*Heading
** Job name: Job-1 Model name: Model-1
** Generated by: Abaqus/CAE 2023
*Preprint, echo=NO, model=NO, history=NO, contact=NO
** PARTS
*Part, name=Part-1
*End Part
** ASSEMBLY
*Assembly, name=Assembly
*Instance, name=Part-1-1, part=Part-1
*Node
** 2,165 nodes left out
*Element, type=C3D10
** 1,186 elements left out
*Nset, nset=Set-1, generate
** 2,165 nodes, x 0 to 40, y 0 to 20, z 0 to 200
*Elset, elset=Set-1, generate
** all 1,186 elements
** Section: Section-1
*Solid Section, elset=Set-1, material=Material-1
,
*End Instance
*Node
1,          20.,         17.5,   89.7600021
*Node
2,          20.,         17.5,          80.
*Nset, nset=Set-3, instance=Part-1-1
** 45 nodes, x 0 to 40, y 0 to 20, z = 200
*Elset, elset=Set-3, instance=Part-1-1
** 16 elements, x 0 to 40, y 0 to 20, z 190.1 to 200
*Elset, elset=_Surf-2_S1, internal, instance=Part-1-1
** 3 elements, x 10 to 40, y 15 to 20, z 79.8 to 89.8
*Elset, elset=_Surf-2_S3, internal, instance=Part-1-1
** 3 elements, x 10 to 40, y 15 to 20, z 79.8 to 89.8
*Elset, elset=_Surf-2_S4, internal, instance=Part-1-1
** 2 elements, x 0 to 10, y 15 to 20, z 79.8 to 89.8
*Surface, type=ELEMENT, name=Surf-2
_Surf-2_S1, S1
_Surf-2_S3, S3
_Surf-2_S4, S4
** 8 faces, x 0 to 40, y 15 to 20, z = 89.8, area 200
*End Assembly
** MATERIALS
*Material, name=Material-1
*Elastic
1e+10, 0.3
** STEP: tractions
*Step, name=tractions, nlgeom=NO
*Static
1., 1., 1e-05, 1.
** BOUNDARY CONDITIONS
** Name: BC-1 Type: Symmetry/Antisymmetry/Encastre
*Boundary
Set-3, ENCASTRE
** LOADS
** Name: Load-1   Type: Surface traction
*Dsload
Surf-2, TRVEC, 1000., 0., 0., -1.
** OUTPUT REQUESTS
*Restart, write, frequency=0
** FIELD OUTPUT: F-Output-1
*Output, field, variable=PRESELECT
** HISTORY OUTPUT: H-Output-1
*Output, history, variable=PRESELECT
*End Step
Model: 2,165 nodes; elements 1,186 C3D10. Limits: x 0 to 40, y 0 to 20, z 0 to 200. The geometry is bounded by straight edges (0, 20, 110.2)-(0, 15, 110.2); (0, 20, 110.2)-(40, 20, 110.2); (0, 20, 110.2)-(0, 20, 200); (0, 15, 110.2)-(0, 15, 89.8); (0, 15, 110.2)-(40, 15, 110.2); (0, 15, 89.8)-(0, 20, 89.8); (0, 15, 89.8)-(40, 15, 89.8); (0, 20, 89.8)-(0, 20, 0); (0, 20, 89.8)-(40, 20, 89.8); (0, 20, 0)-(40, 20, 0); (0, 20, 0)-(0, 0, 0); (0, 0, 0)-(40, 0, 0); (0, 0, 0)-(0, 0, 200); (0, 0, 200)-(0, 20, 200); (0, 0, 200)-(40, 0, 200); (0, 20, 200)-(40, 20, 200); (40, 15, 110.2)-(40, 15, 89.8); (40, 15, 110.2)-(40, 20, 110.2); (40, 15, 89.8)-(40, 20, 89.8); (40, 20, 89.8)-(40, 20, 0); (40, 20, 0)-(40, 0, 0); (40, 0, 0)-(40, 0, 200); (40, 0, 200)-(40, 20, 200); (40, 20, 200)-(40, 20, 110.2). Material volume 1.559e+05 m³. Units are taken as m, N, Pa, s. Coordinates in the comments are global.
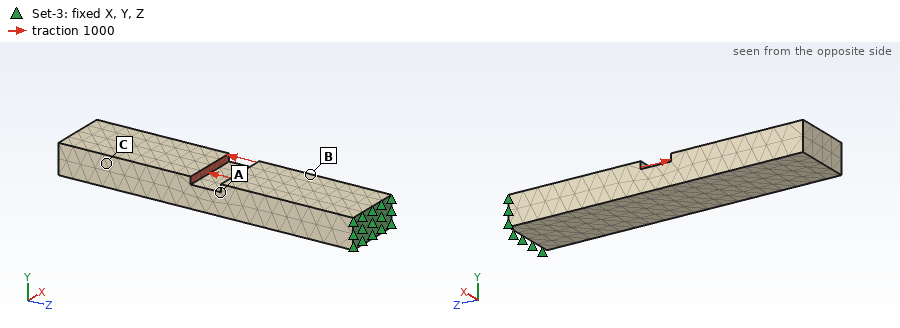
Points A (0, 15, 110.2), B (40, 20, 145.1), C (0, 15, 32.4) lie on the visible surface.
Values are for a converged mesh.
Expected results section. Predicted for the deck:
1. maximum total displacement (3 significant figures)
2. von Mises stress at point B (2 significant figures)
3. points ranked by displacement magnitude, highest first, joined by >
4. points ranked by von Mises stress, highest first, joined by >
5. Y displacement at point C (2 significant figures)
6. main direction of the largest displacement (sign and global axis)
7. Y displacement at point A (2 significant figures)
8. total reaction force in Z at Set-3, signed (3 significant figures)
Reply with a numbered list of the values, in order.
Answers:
1. 1.25e-04 m
2. 810 Pa
3. C > A > B
4. A > B > C
5. -9.3e-05 m
6. -Y
7. -2.2e-05 m
8. 2.00e+05 N
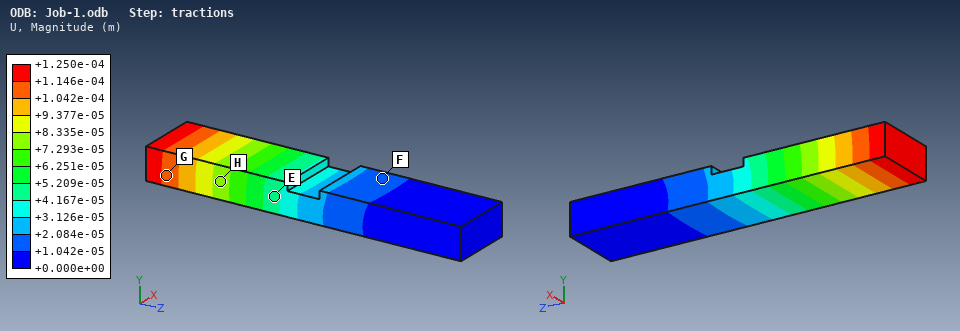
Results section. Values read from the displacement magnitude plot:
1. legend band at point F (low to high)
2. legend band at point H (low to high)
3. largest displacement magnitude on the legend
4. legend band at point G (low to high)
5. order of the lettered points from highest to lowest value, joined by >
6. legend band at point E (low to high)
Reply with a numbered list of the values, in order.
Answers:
1. +1.042e-05 to +2.084e-05 m
2. +7.293e-05 to +8.335e-05 m
3. +1.250e-04 m
4. +1.042e-04 to +1.146e-04 m
5. G > H > E > F
6. +4.167e-05 to +5.209e-05 m
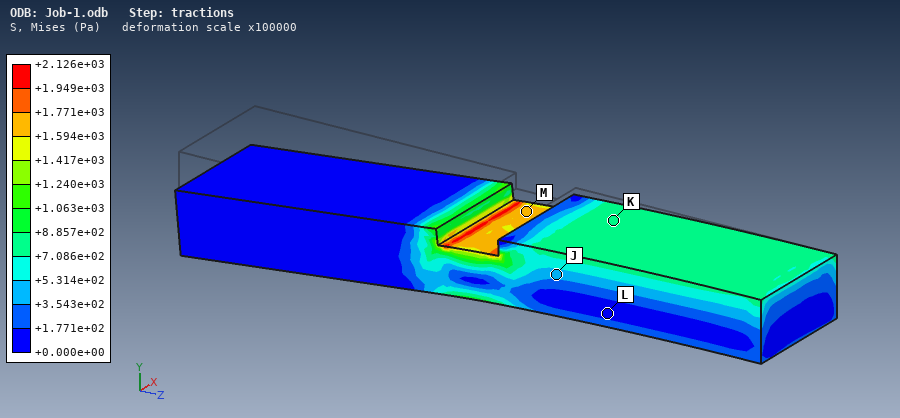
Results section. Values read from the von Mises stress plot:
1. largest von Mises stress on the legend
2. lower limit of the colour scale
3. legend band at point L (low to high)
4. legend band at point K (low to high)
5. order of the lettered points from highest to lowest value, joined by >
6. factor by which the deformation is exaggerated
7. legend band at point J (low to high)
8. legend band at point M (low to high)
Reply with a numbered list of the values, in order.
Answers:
1. +2.126e+03 Pa
2. +0.000e+00 Pa
3. +0.000e+00 to +1.771e+02 Pa
4. +7.086e+02 to +8.857e+02 Pa
5. M > K > J > L
6. 100000
7. +3.543e+02 to +5.314e+02 Pa
8. +1.594e+03 to +1.771e+03 Pa
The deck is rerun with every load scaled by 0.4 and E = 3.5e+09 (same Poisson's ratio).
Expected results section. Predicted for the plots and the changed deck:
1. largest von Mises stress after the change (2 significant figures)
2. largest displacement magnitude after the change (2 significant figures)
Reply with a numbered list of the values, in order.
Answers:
1. 850 Pa
2. 1.4e-04 m
